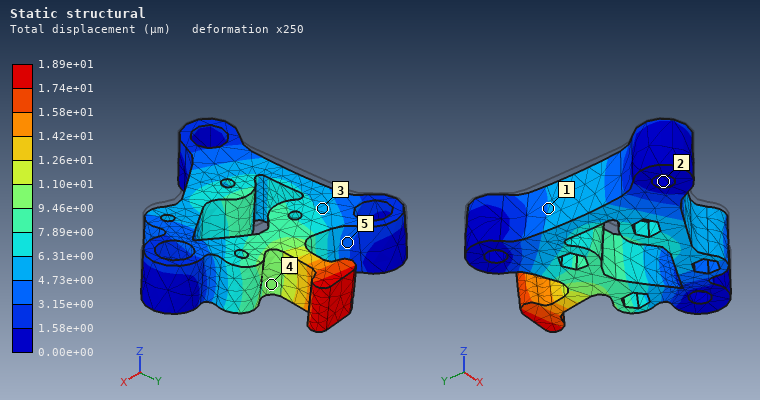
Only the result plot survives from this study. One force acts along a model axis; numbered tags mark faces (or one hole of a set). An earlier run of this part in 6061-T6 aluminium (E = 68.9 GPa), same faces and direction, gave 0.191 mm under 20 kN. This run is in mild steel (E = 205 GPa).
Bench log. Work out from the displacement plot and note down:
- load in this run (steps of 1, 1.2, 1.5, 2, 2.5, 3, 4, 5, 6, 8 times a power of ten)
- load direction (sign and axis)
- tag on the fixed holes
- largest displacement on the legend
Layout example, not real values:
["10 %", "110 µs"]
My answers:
["6 kN", "-Z", "2", "1.89e+01 µm"]
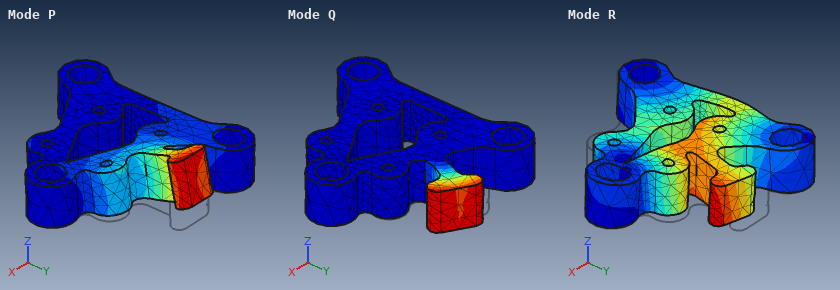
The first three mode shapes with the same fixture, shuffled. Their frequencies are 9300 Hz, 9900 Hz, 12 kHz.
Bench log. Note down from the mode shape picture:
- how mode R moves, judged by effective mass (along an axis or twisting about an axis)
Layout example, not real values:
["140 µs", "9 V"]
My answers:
["along X"]
